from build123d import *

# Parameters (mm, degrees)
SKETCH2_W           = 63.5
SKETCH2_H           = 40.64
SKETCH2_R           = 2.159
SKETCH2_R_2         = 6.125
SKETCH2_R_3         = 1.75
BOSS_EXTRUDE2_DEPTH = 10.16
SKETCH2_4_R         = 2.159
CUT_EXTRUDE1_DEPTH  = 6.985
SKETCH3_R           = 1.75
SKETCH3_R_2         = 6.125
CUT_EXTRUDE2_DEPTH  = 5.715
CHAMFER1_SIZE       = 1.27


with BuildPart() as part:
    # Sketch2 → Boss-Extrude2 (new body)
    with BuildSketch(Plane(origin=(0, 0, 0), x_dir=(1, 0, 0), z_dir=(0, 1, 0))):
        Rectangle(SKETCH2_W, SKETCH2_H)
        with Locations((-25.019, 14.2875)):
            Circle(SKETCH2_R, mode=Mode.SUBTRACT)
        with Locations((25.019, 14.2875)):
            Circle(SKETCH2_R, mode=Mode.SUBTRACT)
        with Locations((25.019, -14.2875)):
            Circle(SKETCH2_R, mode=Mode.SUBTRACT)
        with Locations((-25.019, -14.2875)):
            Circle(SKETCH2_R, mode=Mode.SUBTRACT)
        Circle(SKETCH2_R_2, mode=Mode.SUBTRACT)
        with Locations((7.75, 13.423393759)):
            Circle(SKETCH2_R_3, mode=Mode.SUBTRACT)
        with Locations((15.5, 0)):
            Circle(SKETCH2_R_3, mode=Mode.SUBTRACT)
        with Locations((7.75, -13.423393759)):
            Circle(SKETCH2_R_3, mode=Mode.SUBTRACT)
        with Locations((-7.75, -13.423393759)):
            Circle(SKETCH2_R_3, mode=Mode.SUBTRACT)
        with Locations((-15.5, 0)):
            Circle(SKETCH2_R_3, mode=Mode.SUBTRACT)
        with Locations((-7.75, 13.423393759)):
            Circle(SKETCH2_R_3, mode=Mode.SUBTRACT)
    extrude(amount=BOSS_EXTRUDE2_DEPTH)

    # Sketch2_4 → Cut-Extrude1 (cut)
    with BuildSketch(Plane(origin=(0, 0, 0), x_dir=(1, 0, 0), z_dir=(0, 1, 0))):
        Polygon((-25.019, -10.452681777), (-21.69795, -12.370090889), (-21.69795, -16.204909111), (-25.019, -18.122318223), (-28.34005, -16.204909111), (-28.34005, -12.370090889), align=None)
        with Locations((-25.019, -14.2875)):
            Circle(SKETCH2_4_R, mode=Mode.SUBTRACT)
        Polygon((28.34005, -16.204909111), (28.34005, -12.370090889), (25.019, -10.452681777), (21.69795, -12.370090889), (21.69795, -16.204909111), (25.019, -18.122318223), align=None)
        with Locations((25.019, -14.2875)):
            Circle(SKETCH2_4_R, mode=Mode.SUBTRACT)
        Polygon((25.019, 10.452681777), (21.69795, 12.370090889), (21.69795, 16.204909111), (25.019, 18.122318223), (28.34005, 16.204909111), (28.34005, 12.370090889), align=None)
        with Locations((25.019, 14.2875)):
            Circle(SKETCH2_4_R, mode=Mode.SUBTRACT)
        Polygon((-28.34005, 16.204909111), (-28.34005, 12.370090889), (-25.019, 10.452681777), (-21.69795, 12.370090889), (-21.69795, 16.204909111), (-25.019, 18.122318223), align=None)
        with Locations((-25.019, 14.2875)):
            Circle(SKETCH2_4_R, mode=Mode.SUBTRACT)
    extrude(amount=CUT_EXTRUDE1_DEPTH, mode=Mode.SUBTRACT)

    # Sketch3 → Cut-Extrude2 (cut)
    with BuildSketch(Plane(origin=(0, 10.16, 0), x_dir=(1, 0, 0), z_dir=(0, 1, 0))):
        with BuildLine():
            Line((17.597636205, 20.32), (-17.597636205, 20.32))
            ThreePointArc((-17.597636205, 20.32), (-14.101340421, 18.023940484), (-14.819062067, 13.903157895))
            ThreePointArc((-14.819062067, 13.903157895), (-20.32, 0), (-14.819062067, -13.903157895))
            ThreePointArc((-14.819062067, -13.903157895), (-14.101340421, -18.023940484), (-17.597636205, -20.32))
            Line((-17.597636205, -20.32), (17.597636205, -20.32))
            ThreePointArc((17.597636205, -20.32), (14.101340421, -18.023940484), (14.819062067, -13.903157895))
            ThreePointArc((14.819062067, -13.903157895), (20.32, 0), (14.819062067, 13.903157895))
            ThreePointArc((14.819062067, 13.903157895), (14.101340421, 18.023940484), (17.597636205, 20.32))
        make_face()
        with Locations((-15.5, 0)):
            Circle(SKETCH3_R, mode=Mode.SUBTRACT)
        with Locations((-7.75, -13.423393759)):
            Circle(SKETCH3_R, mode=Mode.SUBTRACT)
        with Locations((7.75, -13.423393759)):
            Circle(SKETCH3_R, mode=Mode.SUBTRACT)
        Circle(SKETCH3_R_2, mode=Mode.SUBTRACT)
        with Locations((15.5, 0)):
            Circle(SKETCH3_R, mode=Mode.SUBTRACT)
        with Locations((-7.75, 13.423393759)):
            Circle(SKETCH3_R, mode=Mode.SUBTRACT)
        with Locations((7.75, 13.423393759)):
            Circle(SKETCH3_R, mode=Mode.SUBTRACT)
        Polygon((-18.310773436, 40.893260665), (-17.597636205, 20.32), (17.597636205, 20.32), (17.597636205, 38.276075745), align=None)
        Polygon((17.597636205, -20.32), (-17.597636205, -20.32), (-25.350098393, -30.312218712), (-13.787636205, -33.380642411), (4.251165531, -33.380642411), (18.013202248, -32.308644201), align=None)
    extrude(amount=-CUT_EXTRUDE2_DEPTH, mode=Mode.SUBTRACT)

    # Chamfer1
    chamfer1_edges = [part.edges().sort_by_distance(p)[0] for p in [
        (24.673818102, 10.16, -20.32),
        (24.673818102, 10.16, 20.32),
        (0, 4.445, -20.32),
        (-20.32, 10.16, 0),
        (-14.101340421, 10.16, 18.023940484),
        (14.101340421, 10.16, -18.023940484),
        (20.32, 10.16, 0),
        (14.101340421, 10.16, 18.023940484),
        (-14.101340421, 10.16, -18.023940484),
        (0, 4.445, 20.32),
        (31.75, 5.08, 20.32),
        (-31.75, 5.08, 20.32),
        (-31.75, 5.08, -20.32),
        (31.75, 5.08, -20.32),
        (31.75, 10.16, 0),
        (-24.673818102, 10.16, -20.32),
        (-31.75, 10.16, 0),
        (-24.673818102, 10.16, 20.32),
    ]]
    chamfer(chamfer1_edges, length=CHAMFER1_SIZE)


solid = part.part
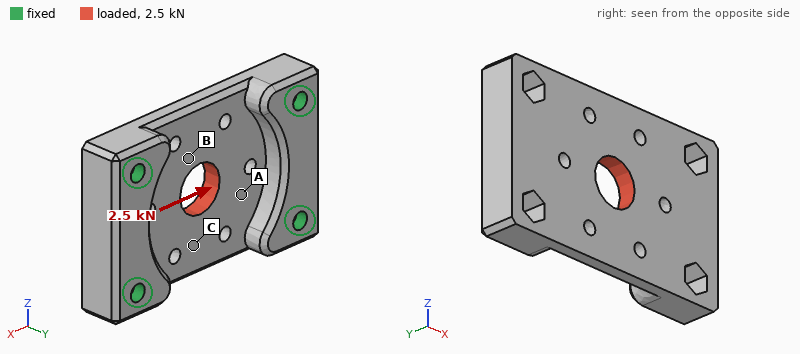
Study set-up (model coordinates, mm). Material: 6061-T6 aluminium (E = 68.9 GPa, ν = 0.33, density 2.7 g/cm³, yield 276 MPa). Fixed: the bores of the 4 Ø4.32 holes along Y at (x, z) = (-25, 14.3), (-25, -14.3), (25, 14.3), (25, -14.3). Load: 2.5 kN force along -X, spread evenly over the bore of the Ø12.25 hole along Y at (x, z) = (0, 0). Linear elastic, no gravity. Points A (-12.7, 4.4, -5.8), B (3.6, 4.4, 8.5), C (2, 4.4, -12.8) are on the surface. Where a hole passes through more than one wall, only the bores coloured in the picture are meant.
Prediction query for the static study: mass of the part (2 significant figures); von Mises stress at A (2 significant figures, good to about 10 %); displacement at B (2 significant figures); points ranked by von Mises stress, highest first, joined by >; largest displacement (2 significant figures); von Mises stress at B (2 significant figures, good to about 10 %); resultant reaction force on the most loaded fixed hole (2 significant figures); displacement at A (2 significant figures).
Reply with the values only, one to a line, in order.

43 g
22 MPa
9.6 µm
A > B > C
11 µm
15 MPa
630 N
9.3 µm
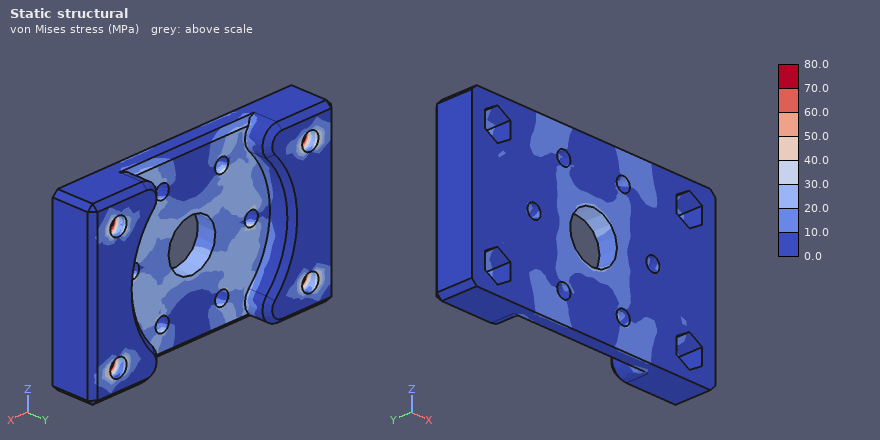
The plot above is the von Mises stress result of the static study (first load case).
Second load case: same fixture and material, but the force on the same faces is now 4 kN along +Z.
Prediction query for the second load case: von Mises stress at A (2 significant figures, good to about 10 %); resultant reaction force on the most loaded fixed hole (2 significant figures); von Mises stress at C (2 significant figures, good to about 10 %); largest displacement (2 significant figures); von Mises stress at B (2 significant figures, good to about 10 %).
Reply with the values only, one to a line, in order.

27 MPa
1.2 kN
19 MPa
17 µm
21 MPa
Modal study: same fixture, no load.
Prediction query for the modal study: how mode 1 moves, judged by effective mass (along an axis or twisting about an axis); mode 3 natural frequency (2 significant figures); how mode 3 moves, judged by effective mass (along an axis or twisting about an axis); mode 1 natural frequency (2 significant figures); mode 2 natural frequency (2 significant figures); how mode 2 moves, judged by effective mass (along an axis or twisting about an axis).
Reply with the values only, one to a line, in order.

along Y
16 kHz
twisting about X
12 kHz
14 kHz
along X
